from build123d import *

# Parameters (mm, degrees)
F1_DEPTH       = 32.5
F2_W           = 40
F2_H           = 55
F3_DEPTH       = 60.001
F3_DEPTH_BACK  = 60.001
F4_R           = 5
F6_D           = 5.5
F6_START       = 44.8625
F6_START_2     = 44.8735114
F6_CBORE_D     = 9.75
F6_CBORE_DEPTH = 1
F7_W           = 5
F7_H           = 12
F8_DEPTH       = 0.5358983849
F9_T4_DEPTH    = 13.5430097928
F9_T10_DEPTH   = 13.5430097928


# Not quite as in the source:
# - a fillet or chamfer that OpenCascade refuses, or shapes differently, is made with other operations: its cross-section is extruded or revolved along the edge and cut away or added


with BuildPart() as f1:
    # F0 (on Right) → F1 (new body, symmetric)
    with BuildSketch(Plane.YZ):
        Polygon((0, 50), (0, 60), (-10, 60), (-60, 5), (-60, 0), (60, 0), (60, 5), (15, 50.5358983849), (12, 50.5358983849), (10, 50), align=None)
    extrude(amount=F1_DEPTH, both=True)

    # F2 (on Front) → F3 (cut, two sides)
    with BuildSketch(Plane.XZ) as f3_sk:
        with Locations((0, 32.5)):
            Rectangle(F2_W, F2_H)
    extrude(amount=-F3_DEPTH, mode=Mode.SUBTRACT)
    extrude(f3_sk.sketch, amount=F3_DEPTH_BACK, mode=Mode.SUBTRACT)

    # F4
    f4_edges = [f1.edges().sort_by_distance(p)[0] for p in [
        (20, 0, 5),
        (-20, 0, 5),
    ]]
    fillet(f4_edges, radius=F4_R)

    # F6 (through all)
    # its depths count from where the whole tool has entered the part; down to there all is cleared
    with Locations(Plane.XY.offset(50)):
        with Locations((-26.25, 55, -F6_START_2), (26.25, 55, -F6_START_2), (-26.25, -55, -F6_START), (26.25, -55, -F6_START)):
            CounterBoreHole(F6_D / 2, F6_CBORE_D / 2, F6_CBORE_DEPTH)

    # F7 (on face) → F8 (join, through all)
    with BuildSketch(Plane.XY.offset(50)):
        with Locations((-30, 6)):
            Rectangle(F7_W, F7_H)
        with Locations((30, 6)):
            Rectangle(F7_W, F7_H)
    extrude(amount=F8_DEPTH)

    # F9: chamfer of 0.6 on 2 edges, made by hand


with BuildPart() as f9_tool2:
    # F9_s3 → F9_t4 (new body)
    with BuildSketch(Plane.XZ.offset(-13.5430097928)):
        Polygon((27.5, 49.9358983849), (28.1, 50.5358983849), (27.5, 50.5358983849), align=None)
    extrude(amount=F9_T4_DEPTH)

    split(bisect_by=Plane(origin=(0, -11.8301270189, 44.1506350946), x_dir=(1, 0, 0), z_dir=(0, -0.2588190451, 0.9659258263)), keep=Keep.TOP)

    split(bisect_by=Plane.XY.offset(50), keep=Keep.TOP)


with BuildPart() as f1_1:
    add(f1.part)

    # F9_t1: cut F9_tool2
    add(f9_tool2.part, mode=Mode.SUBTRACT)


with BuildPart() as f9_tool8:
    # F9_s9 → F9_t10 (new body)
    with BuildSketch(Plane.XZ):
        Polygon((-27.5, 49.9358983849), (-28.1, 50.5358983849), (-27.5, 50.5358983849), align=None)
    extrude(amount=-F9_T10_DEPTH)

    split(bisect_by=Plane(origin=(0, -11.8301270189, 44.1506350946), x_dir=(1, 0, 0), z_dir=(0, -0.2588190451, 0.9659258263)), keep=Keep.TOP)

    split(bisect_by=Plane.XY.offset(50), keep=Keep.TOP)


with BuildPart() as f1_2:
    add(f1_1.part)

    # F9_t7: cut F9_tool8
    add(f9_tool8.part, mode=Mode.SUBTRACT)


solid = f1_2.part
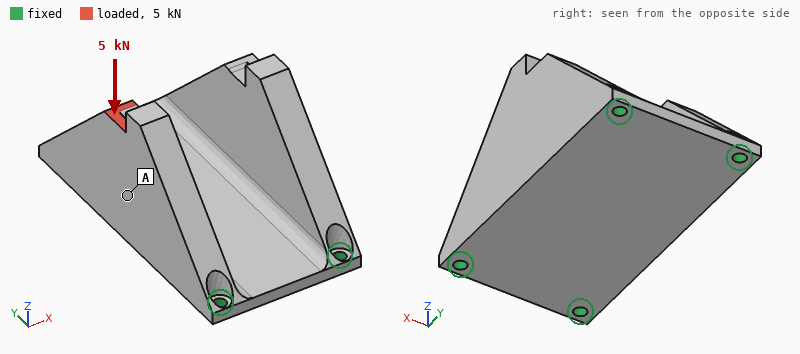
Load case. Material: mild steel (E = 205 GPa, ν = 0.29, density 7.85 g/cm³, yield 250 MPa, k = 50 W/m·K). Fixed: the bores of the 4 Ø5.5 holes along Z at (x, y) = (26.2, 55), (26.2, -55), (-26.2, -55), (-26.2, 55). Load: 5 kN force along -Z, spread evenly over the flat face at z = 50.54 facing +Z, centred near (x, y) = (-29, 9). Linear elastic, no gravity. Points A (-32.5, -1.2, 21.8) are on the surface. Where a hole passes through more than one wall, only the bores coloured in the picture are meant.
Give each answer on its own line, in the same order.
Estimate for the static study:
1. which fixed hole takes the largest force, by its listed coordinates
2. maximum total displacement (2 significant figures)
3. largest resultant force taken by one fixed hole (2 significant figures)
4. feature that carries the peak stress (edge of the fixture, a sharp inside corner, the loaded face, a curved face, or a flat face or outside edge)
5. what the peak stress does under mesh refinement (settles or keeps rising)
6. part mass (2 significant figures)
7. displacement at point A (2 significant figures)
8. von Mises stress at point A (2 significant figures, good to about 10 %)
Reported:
(-26.2, 55)
34 µm
3.7 kN
edge of the fixture
keeps rising
1.0 kg
15 µm
9.3 MPa
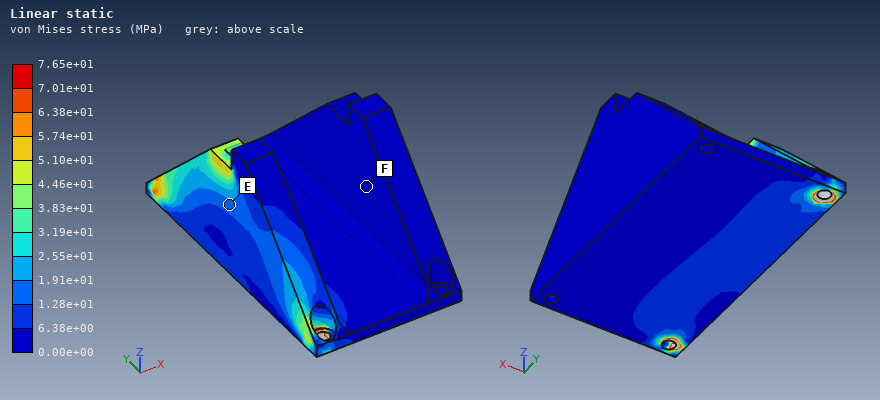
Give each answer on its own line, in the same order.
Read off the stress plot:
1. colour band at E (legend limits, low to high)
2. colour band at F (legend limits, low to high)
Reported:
1.28e+01 to 1.91e+01 MPa
0.00e+00 to 6.38e+00 MPa
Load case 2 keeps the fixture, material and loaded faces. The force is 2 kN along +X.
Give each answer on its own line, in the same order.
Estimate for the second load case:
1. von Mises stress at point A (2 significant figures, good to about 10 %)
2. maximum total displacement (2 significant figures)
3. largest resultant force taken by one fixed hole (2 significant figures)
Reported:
27 MPa
0.15 mm
1.3 kN
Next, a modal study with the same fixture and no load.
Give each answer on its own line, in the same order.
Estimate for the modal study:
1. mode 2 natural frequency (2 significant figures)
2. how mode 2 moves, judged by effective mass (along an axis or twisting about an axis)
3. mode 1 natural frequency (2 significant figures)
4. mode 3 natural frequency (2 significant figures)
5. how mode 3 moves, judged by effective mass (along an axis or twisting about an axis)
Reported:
2400 Hz
along X
1800 Hz
5800 Hz
along Z
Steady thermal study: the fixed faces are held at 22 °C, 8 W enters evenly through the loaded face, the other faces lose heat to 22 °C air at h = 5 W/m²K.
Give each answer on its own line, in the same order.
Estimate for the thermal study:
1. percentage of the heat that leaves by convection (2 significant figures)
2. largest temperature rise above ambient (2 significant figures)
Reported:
10 %
25 K
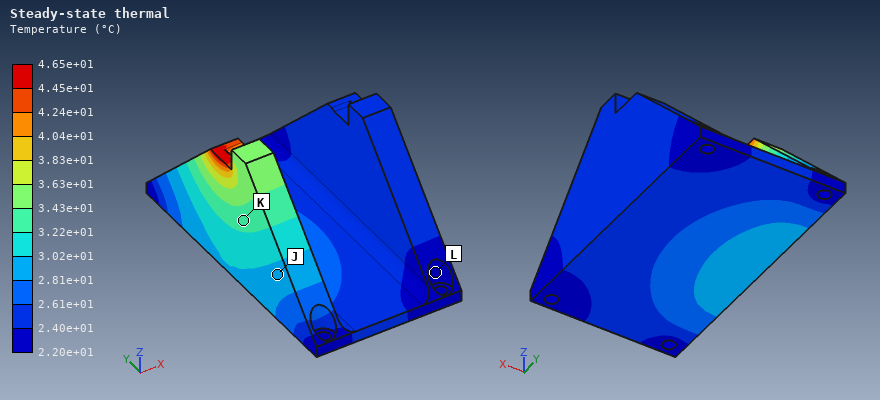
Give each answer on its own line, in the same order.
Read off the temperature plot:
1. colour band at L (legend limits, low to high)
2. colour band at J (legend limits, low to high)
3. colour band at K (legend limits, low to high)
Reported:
2.20e+01 to 2.40e+01 °C
2.81e+01 to 3.02e+01 °C
3.22e+01 to 3.43e+01 °C
